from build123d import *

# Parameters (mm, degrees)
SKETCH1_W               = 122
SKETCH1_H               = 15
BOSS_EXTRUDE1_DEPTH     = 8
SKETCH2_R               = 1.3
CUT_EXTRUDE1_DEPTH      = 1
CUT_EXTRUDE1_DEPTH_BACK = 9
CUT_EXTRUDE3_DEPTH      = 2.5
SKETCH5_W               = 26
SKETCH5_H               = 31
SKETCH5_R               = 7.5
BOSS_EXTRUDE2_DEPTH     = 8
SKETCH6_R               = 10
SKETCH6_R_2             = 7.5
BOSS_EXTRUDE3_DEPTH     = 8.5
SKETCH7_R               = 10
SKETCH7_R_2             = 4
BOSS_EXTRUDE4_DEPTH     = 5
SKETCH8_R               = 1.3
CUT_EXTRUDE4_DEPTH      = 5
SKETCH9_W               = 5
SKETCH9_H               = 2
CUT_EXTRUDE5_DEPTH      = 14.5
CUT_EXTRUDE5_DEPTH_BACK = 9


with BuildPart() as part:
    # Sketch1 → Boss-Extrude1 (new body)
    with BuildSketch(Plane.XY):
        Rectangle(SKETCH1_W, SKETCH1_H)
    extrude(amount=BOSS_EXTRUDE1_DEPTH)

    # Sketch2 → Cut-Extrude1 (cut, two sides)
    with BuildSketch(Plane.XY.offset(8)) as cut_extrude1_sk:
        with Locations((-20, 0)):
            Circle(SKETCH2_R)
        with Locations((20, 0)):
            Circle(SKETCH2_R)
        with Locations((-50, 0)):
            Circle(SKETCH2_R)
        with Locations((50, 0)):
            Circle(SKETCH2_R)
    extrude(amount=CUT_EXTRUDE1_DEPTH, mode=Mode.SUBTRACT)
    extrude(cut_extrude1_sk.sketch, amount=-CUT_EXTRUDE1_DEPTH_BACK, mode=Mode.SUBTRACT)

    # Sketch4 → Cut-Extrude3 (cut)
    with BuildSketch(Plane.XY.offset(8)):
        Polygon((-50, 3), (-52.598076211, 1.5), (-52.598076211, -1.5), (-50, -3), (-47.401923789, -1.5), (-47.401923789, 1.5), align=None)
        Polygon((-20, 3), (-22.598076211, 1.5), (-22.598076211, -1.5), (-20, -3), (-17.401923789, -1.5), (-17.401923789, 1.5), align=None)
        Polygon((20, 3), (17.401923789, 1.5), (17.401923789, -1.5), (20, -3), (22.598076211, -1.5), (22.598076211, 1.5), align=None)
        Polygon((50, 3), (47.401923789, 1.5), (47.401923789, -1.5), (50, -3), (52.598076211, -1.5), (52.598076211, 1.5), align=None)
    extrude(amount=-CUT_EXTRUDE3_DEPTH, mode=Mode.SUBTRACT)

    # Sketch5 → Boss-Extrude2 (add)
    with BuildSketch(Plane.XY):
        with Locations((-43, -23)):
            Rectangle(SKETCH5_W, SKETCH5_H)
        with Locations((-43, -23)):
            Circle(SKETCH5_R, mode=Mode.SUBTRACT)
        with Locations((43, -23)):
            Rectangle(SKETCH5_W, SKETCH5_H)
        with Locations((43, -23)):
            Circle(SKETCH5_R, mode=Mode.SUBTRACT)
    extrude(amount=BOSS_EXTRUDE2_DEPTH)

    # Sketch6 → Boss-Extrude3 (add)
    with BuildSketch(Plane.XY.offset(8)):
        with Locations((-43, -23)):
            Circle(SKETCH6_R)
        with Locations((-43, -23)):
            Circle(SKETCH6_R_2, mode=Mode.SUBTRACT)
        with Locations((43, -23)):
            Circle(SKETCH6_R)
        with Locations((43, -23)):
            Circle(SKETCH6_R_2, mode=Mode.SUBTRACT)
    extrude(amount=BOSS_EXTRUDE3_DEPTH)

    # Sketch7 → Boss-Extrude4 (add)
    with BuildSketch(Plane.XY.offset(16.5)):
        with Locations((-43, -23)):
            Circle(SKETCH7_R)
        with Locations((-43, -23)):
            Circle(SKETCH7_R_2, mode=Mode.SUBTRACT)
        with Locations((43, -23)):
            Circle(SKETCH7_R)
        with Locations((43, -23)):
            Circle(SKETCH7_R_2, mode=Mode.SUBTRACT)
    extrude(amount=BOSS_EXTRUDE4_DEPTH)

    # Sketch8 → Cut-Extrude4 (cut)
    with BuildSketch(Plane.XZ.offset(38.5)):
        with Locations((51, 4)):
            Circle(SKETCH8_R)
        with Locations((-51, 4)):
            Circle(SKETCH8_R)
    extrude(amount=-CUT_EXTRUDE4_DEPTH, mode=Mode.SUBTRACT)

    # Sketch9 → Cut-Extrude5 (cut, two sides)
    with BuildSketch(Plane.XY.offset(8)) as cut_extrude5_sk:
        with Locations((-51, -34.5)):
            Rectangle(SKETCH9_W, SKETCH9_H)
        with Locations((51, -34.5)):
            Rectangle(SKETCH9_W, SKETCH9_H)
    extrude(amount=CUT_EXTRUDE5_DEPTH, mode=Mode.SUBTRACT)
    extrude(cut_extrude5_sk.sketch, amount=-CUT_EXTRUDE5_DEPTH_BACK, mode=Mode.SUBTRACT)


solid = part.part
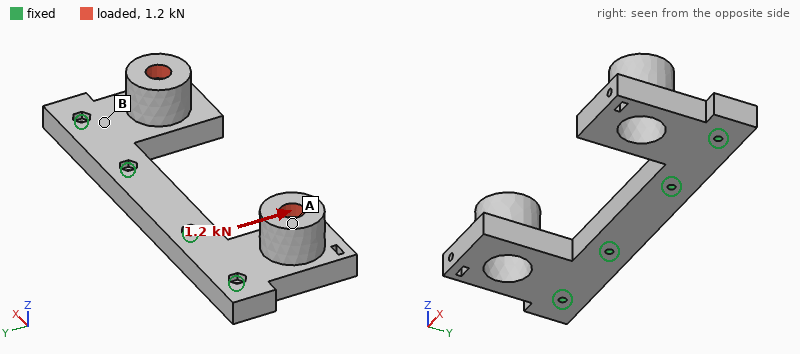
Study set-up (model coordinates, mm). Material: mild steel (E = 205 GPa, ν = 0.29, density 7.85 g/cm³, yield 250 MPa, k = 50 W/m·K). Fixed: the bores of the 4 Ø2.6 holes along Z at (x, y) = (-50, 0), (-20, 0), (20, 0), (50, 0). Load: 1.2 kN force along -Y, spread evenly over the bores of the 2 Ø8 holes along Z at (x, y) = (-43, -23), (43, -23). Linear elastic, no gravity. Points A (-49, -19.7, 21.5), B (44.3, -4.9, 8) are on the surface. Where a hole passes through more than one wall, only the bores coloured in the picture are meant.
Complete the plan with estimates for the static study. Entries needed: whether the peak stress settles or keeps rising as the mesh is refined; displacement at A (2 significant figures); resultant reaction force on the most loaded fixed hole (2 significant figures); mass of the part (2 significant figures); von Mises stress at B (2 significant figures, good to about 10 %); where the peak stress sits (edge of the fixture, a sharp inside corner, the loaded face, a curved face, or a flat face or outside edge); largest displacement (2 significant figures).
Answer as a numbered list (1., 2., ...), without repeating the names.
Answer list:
1. keeps rising
2. 29 µm
3. 440 N
4. 230 g
5. 28 MPa
6. edge of the fixture
7. 41 µm
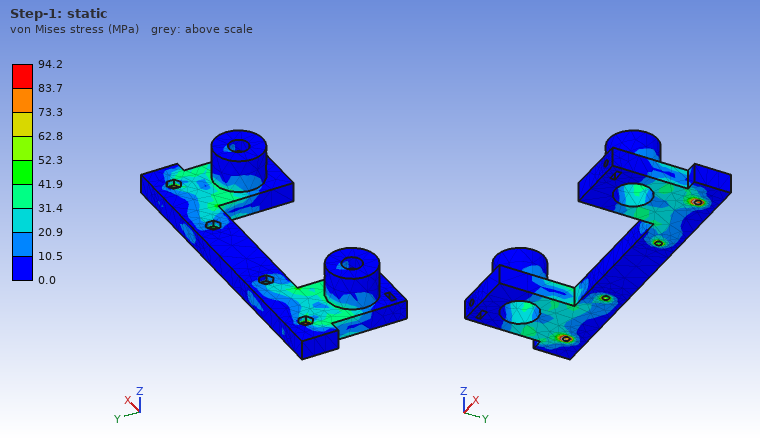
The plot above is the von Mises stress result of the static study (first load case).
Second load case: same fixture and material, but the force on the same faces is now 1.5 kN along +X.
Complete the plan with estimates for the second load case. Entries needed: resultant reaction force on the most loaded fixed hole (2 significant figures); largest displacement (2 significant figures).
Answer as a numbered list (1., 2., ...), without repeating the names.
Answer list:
1. 920 N
2. 19 µm
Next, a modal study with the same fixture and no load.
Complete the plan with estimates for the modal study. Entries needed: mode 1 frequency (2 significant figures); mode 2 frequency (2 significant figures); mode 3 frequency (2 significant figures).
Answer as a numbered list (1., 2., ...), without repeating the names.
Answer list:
1. 2800 Hz
2. 2800 Hz
3. 7100 Hz
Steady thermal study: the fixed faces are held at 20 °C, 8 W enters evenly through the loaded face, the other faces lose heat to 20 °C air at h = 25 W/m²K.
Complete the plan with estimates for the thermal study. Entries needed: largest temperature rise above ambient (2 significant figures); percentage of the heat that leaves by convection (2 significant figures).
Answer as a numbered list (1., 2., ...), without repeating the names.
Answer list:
1. 16 K
2. 25 %
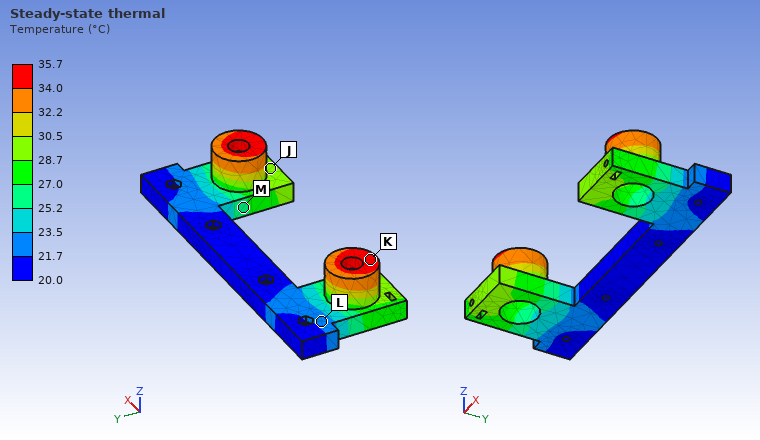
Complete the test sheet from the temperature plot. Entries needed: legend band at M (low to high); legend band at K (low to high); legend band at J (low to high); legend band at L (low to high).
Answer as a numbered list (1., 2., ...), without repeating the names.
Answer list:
1. 25.2 to 27.0 °C
2. 34.0 to 35.7 °C
3. 28.7 to 30.5 °C
4. 21.7 to 23.5 °C
